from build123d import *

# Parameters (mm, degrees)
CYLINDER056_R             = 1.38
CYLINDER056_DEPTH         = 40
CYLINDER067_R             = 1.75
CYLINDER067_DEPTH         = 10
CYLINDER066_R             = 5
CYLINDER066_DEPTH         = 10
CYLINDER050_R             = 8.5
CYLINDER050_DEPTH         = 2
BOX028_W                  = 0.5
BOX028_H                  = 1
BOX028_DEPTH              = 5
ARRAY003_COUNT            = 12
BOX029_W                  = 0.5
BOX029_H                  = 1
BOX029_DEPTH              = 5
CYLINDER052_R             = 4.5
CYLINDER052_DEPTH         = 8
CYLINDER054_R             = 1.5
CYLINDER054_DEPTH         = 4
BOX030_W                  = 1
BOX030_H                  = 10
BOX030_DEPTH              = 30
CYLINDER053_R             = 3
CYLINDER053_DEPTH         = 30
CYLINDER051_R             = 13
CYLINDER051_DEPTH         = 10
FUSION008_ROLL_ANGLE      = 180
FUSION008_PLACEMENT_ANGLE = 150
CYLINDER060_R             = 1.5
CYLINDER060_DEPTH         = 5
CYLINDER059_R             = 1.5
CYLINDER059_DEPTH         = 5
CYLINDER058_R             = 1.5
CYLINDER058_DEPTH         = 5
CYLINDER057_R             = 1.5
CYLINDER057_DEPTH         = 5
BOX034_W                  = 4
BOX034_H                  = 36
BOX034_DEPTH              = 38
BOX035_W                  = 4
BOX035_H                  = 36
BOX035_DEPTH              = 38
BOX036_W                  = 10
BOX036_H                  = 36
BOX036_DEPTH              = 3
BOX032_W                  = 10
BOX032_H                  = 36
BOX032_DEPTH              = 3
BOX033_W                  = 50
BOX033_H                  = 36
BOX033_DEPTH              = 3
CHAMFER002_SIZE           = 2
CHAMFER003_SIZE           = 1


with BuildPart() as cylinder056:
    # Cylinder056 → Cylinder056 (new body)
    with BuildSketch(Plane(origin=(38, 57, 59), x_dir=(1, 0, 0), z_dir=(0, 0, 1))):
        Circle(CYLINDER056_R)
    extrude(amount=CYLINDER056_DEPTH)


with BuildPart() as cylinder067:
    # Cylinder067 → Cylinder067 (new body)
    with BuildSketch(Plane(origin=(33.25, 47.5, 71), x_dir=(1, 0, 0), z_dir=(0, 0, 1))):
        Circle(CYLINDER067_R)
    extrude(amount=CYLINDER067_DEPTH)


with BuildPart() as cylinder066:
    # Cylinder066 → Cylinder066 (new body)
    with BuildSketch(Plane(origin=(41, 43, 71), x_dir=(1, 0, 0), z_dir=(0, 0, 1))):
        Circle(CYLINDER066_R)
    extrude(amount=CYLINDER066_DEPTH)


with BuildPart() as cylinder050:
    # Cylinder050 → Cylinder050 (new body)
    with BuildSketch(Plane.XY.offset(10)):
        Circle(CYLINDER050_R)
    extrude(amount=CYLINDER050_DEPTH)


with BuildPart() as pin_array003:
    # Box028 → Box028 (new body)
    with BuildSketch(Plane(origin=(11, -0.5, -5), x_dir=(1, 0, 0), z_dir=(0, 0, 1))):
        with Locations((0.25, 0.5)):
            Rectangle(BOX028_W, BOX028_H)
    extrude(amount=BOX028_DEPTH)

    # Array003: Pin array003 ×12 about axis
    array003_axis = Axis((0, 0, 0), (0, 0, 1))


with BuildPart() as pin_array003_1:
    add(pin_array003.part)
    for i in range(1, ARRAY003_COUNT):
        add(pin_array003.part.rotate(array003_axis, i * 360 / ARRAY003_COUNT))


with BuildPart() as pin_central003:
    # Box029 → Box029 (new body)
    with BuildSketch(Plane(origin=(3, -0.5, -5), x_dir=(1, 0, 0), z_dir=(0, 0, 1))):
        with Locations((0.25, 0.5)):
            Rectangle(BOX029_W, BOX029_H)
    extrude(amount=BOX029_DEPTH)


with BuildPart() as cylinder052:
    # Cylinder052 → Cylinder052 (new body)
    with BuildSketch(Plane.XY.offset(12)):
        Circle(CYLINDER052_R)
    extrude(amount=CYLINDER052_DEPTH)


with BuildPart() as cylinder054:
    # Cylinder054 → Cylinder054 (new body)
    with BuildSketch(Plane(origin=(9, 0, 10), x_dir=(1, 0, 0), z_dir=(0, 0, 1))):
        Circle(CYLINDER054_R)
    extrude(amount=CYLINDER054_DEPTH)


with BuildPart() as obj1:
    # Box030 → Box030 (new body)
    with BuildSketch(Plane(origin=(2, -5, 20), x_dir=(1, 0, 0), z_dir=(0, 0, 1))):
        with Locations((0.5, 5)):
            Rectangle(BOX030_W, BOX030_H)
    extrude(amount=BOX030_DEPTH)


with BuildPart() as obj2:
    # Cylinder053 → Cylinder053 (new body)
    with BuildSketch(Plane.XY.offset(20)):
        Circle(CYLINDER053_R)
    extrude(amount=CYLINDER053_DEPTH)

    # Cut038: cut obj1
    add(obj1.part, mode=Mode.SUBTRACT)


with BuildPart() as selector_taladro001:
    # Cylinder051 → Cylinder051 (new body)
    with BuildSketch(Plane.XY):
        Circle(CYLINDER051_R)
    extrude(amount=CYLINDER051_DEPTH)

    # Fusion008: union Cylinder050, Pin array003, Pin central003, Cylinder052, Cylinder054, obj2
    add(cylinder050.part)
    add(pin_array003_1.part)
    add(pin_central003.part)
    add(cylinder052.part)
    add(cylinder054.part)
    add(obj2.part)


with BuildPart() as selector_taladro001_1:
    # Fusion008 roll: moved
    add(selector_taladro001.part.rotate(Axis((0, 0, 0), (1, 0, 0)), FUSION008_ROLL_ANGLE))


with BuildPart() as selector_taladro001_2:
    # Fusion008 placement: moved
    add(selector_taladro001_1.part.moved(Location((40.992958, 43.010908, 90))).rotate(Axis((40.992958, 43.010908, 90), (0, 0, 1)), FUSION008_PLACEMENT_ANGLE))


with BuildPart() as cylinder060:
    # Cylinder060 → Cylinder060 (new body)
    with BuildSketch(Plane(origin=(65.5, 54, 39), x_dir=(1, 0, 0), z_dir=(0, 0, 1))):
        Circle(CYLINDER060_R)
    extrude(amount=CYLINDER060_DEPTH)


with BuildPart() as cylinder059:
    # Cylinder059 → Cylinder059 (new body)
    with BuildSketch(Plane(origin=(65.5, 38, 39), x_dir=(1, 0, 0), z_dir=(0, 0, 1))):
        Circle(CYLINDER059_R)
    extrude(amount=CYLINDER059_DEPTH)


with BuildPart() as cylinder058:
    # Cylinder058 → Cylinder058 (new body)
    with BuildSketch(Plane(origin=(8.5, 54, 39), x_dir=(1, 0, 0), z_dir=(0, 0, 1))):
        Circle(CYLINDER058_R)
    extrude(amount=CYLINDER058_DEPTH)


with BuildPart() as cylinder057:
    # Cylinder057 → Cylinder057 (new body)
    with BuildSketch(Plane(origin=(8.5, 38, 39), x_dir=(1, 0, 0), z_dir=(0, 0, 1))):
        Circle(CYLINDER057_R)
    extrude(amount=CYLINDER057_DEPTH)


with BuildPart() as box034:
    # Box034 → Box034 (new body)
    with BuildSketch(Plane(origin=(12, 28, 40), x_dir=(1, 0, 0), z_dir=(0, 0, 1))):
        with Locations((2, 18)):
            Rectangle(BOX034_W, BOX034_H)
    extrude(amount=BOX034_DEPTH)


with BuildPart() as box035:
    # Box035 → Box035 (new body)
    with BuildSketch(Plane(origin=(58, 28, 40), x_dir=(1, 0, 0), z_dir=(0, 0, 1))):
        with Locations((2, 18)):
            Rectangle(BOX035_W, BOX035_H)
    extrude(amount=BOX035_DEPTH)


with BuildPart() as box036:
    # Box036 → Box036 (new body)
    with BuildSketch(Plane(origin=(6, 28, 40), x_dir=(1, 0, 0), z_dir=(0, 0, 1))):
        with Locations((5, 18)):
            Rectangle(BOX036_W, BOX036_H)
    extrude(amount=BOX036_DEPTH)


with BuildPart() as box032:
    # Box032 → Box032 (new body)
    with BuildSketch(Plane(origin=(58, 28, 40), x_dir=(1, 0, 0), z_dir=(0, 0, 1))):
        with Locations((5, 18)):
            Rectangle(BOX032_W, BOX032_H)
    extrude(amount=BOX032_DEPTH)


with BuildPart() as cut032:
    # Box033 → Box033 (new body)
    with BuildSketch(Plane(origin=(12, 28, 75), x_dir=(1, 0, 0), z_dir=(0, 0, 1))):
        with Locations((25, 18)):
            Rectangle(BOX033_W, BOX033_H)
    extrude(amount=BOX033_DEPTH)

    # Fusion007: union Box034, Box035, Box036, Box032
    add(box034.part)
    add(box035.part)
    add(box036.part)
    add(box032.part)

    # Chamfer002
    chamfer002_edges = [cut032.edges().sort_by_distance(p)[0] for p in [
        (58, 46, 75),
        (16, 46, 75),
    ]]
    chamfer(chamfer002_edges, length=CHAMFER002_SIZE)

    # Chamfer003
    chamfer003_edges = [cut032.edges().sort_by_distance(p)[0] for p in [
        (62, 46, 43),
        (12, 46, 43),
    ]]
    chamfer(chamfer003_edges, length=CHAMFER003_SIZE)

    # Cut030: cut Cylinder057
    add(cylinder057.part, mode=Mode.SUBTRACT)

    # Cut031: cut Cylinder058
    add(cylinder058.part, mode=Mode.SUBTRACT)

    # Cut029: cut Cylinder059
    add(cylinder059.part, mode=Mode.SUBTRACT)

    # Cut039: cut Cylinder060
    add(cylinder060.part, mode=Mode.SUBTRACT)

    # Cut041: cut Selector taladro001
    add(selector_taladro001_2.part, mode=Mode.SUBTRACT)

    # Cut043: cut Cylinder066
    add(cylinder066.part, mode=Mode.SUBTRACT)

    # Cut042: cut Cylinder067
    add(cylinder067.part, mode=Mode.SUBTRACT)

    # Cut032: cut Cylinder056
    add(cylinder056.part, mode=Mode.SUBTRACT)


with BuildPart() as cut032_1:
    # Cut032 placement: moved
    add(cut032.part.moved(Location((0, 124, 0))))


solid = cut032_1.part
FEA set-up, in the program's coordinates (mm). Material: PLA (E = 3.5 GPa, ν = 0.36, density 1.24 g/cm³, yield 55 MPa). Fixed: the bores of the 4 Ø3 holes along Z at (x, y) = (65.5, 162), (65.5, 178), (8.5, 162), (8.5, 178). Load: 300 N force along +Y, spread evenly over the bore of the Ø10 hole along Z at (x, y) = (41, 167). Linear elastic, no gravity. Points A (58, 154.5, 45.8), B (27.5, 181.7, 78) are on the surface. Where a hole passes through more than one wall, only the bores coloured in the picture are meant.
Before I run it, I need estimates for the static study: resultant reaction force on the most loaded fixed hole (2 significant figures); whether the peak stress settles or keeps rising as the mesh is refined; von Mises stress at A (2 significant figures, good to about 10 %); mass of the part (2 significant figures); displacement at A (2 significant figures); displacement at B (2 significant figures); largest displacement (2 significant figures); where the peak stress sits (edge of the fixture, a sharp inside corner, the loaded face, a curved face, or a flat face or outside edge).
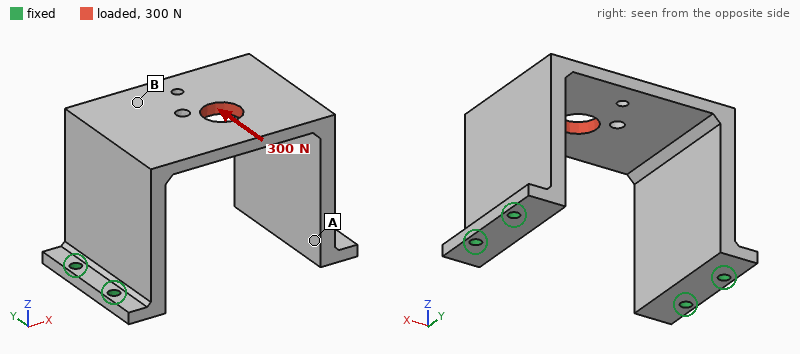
340 N
keeps rising
8.0 MPa
21 g
0.22 mm
0.42 mm
0.55 mm
edge of the fixture
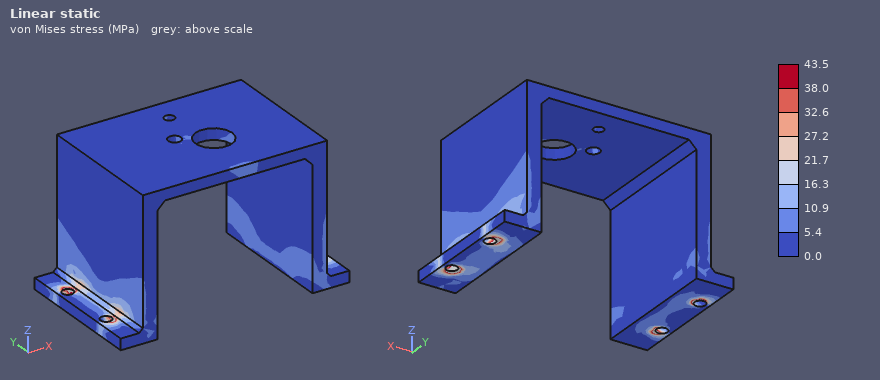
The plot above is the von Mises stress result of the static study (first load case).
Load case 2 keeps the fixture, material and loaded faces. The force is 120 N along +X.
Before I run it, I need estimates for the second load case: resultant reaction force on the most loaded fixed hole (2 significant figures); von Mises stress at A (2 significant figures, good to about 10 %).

48 N
6.3 MPa
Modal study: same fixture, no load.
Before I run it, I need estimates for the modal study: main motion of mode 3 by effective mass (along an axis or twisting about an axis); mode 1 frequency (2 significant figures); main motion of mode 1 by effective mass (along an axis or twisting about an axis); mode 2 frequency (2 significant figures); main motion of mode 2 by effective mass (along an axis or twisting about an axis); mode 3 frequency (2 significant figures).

twisting about Z
600 Hz
along X
1300 Hz
along Y
1400 Hz
